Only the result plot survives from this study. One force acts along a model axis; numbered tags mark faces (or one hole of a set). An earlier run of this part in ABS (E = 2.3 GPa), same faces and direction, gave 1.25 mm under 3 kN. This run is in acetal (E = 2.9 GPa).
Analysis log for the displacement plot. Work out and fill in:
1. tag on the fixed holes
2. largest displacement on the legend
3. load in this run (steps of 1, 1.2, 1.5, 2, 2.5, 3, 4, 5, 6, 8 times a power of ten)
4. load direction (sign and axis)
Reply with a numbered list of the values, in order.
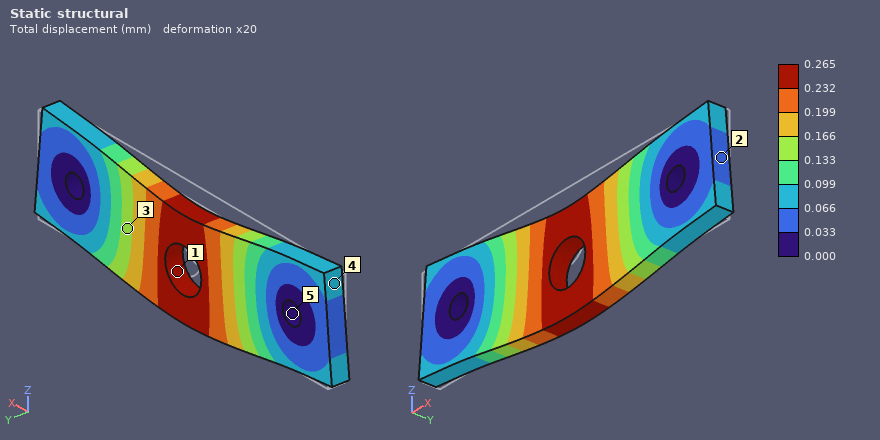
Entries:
1. 5
2. 0.265 mm
3. 800 N
4. -Z
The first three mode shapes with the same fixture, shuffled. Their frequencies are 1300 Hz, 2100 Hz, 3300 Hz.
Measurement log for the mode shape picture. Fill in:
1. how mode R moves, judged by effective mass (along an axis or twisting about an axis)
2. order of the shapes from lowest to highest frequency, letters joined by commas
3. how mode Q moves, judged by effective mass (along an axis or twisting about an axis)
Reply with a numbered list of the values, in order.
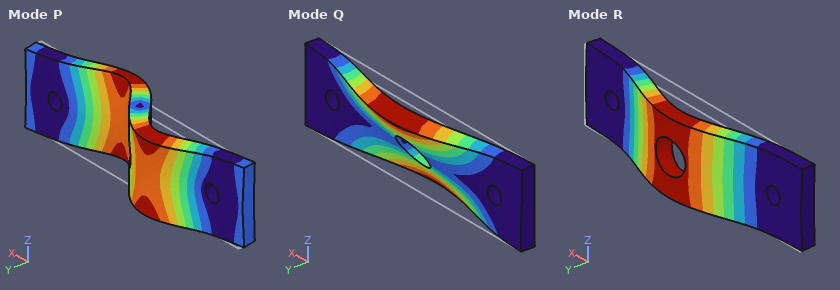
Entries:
1. along Y
2. R, Q, P
3. twisting about X
